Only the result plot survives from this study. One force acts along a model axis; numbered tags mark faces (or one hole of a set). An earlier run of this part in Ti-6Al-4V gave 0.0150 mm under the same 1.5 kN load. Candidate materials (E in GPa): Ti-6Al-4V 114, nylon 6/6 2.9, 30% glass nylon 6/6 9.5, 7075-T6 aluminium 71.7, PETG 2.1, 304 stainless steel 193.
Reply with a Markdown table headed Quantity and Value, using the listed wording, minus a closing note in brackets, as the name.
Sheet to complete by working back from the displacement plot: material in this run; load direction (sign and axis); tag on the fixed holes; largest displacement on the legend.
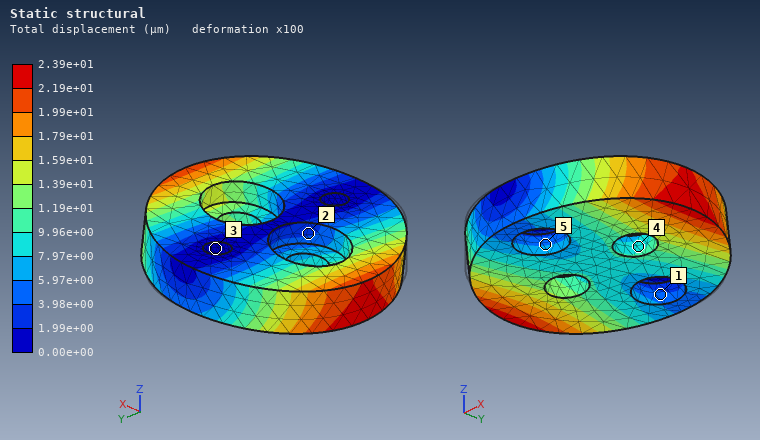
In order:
| Quantity | Value |
|---|---|
| material in this run | 7075-T6 aluminium |
| load direction | +X |
| tag on the fixed holes | 3 |
| largest displacement on the legend | 2.39e+01 µm |
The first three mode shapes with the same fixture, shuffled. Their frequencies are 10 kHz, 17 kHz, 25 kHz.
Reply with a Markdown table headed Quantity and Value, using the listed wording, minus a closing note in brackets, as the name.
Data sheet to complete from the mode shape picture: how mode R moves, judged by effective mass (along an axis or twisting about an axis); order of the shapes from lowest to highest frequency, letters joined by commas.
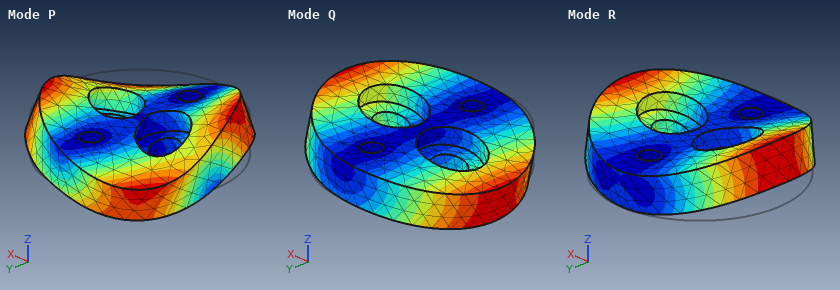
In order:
| Quantity | Value |
|---|---|
| how mode R moves, judged by effective mass | along Z |
| order of the shapes from lowest to highest frequency, letters joined by commas | Q, R, P |
